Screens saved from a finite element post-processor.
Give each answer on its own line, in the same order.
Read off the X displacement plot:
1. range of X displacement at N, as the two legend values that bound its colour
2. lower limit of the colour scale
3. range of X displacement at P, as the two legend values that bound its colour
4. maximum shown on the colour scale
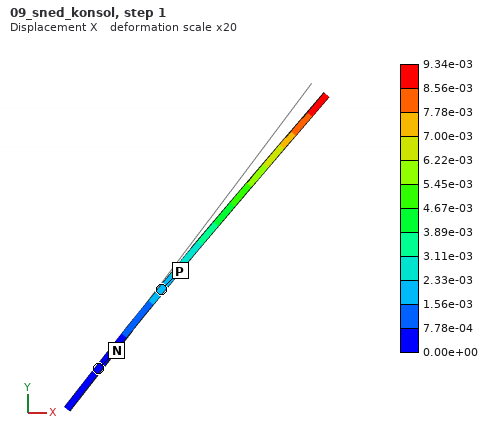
0.00e+00 to 7.78e-04
0.00e+00
1.56e-03 to 2.33e-03
9.34e-03
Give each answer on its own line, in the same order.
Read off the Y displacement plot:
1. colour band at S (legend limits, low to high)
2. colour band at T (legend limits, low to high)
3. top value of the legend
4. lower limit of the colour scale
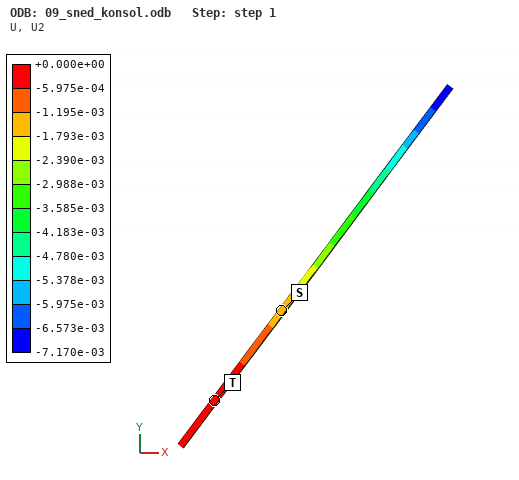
-1.793e-03 to -1.195e-03
-5.975e-04 to +0.000e+00
+0.000e+00
-7.170e-03
